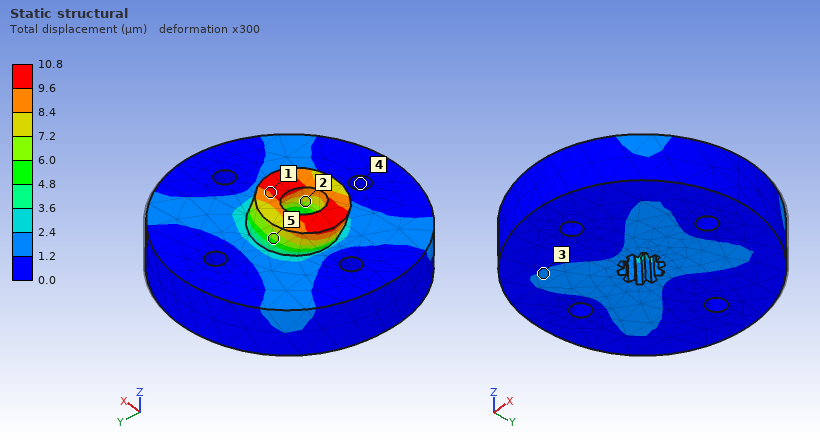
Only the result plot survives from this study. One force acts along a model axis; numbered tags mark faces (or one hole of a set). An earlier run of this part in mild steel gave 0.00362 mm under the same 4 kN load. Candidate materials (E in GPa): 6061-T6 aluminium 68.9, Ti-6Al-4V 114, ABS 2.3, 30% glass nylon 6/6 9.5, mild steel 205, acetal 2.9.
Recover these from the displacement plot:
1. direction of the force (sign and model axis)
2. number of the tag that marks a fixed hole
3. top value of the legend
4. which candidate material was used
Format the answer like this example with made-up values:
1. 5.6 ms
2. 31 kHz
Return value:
1. -X
2. 4
3. 10.8 µm
4. 6061-T6 aluminium
